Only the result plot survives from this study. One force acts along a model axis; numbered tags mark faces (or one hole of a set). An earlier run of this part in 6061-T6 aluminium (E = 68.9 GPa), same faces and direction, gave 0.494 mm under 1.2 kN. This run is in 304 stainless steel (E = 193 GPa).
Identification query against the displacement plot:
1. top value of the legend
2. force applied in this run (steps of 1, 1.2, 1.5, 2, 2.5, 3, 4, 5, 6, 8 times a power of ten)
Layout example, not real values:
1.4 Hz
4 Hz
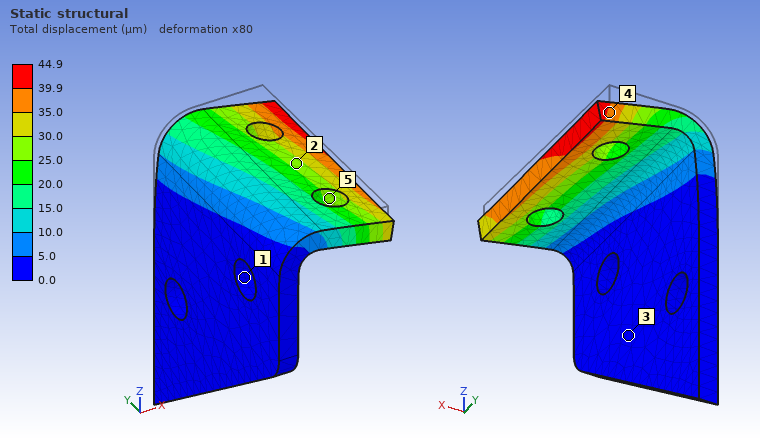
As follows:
44.9 µm
300 N
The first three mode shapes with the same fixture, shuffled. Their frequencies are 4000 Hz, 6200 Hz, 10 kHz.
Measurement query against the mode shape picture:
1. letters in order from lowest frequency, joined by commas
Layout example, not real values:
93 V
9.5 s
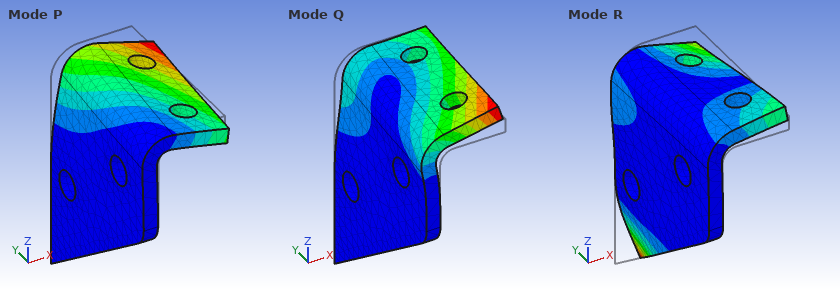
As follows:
P, Q, R
